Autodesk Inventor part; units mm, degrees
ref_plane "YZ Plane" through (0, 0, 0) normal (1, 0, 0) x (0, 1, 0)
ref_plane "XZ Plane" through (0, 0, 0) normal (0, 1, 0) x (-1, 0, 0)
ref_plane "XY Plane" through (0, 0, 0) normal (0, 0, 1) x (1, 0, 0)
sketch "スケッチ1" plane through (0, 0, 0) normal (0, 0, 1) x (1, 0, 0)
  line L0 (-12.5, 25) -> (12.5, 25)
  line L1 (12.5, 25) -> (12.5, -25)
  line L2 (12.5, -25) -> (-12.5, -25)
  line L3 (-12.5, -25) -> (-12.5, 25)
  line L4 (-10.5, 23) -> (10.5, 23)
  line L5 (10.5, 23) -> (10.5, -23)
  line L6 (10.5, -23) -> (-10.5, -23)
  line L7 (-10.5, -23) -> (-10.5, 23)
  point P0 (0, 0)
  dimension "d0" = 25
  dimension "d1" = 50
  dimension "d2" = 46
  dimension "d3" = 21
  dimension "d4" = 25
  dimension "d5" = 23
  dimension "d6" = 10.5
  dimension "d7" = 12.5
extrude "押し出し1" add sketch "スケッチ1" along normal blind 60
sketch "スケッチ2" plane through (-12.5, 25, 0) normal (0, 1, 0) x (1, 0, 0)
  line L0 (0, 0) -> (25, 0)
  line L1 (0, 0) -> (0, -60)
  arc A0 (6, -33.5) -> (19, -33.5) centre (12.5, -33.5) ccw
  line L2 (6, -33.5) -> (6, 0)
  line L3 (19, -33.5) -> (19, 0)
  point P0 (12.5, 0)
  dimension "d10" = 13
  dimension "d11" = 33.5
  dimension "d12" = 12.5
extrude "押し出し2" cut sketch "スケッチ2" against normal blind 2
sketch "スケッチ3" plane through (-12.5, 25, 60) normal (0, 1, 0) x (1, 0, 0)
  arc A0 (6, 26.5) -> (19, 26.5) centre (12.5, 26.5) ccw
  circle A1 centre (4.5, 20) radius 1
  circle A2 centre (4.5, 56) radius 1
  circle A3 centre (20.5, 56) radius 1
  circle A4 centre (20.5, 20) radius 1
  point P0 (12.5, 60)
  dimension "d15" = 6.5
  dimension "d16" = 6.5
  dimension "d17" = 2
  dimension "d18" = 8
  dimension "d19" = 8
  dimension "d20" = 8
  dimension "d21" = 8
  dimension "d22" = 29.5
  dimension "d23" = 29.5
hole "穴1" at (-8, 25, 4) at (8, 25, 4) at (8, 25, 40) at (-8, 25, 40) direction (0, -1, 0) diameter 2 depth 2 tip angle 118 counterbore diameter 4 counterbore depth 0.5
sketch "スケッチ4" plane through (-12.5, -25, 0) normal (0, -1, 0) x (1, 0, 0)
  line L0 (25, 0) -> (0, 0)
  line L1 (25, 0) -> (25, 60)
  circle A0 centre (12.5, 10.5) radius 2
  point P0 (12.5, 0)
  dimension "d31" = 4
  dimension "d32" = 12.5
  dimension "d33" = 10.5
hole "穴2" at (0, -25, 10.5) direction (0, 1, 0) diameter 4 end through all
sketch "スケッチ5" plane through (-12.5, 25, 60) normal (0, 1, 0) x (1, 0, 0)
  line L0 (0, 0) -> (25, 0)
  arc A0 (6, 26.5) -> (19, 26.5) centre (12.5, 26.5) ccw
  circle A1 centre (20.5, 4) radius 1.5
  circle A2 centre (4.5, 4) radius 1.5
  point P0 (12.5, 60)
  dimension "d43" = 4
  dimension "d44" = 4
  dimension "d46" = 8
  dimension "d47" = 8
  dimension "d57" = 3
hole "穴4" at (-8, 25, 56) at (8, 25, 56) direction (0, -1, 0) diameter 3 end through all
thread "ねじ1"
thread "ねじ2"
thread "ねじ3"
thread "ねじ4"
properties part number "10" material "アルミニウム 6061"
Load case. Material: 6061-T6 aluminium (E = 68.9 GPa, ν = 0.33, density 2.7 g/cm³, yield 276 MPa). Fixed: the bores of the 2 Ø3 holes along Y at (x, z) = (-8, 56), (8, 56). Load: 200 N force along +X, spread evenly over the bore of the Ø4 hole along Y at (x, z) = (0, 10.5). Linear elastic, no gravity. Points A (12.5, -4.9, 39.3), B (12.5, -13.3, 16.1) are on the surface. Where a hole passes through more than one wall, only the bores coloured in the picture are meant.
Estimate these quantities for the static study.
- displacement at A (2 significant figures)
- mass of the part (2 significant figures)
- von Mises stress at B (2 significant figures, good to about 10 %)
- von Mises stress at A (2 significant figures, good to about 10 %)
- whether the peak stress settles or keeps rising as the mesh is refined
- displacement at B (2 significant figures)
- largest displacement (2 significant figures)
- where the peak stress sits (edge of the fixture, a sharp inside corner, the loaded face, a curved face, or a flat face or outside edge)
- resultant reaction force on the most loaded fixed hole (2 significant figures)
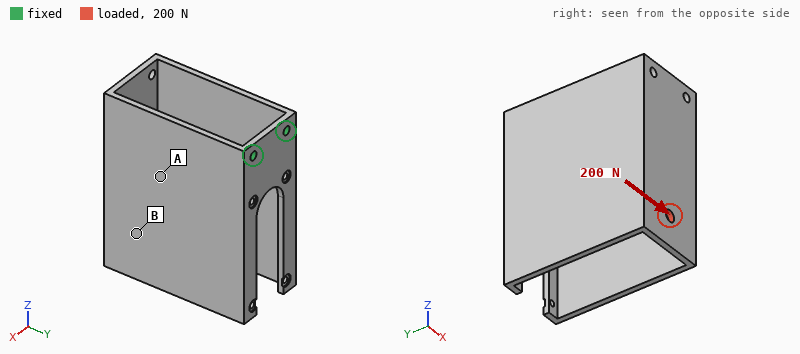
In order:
0.47 mm
43 g
44 MPa
20 MPa
keeps rising
0.69 mm
0.83 mm
edge of the fixture
630 N
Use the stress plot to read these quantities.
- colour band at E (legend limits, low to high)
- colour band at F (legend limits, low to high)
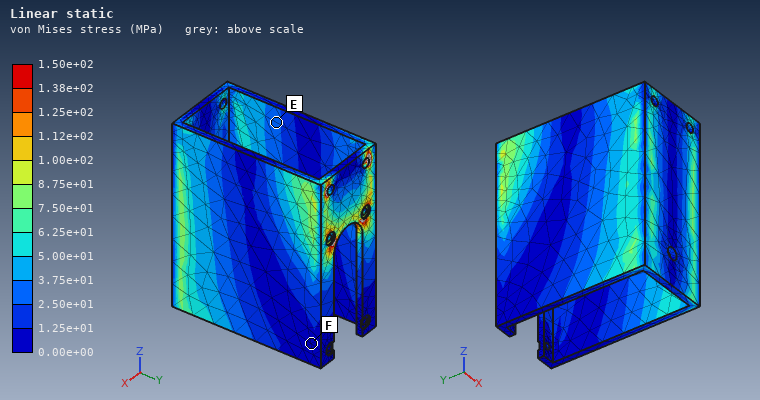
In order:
2.50e+01 to 3.75e+01 MPa
0.00e+00 to 1.25e+01 MPa
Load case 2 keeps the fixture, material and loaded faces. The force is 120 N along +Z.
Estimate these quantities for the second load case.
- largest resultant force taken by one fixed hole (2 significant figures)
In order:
60 N
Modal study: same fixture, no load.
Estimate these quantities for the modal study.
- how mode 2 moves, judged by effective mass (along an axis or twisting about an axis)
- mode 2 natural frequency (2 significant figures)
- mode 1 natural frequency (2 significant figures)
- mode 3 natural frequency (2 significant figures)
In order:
along X
570 Hz
490 Hz
1100 Hz
